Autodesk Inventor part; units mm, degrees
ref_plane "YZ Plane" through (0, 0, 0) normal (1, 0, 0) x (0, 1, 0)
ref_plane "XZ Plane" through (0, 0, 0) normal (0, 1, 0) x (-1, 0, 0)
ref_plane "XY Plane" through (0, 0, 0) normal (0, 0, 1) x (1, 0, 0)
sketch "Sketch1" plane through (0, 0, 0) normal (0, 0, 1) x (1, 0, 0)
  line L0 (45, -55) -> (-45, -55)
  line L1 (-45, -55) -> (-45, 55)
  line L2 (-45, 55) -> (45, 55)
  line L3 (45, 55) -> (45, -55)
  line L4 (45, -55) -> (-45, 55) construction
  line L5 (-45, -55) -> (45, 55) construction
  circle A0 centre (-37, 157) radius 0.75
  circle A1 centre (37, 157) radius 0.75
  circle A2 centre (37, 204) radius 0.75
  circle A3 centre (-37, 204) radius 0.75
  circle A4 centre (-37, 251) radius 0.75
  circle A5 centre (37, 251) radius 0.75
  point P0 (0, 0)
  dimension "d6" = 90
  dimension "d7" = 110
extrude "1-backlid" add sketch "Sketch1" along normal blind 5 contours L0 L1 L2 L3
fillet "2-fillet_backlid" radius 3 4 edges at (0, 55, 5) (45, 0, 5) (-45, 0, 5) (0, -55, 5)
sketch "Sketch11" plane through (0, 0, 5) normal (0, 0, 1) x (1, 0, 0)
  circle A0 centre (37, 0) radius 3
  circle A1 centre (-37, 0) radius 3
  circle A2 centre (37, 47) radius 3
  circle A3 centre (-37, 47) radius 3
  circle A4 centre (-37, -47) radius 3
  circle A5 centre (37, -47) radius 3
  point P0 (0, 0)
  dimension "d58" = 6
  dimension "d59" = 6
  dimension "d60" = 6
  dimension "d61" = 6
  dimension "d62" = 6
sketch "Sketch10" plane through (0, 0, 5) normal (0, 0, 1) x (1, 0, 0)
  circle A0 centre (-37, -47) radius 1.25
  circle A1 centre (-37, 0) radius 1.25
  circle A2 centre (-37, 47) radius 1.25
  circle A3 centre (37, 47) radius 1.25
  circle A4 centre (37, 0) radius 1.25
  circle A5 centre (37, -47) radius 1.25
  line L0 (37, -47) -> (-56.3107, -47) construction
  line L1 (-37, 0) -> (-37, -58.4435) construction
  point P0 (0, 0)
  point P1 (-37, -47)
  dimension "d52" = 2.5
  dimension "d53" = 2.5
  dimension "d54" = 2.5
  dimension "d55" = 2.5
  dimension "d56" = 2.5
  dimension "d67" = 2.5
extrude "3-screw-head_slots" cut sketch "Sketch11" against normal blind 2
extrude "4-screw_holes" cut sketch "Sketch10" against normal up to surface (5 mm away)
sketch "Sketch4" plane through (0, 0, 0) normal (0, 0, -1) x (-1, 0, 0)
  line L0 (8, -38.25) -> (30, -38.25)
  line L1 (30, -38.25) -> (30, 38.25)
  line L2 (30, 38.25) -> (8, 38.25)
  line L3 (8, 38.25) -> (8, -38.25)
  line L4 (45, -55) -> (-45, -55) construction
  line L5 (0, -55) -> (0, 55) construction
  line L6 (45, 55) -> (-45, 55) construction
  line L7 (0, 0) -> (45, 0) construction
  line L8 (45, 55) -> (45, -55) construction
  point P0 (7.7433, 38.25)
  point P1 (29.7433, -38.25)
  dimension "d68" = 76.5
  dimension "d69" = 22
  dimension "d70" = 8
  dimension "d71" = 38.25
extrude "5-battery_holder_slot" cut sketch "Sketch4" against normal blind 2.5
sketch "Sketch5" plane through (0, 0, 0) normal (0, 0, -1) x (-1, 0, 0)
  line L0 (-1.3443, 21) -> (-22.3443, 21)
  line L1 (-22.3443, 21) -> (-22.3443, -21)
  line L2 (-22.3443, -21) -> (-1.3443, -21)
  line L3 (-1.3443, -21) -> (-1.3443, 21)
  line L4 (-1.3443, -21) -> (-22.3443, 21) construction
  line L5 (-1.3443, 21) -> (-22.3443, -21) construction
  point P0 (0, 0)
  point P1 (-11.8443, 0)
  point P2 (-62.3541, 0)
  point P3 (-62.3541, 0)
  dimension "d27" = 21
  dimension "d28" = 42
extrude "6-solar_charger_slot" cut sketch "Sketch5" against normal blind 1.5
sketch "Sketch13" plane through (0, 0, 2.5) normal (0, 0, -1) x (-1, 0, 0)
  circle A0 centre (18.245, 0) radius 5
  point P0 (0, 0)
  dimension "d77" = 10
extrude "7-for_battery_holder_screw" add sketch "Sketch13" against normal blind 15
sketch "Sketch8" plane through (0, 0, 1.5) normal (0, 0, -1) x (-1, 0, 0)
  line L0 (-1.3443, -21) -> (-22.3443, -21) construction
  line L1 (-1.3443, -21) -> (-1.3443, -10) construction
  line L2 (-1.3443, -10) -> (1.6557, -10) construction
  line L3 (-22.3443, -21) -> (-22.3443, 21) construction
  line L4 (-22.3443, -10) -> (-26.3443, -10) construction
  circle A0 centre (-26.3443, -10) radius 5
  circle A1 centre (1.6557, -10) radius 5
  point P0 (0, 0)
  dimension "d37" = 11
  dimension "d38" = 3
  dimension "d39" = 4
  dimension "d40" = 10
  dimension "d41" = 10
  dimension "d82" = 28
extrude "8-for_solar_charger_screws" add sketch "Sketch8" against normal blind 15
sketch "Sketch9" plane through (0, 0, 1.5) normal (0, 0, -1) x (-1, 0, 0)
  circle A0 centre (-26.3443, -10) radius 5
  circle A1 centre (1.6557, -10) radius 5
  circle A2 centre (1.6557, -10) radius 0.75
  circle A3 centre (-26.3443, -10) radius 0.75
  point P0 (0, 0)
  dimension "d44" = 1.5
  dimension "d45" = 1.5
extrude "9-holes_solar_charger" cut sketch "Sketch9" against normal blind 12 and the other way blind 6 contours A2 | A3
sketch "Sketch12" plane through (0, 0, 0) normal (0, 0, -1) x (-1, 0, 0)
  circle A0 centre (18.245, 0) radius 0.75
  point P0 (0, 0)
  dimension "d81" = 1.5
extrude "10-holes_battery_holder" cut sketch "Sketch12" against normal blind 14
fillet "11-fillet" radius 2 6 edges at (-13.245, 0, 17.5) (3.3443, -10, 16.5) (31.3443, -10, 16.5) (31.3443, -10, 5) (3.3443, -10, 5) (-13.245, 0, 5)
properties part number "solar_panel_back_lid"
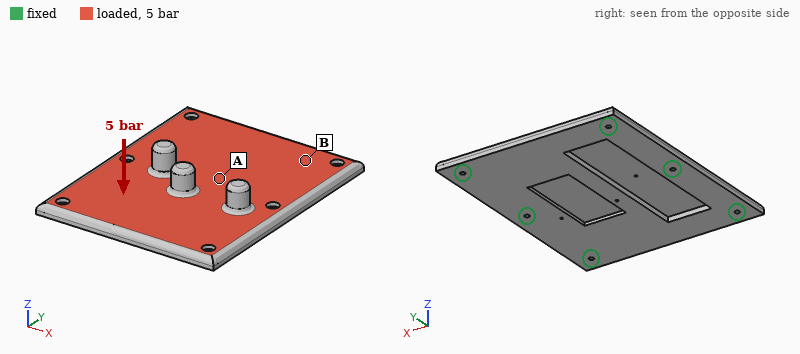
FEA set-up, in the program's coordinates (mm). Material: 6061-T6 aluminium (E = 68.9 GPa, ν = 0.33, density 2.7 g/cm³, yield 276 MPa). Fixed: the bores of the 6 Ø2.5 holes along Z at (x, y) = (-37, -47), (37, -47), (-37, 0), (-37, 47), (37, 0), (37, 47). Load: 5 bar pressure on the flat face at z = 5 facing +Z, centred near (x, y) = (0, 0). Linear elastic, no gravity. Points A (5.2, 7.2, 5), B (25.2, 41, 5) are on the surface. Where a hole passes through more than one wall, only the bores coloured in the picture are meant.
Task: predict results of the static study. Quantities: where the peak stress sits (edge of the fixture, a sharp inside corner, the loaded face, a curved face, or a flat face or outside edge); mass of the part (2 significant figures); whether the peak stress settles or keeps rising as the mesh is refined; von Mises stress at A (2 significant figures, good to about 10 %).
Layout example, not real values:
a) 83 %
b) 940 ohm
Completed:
a) edge of the fixture
b) 120 g
c) keeps rising
d) 46 MPa
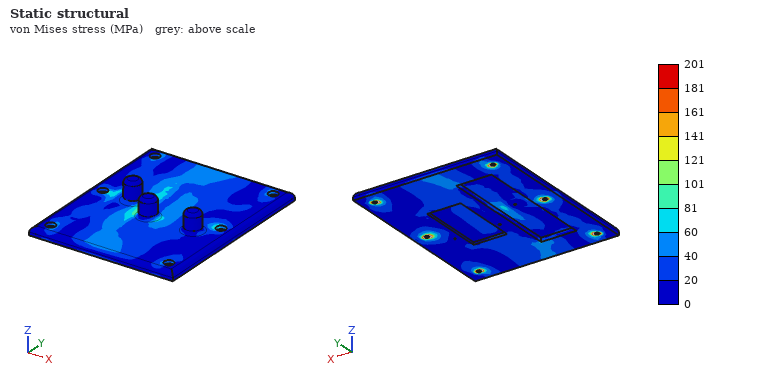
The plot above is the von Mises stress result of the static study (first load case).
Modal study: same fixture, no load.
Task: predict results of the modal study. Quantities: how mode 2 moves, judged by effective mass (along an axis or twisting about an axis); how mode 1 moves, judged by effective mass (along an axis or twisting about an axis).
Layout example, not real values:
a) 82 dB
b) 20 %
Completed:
a) twisting about X
b) along Z
